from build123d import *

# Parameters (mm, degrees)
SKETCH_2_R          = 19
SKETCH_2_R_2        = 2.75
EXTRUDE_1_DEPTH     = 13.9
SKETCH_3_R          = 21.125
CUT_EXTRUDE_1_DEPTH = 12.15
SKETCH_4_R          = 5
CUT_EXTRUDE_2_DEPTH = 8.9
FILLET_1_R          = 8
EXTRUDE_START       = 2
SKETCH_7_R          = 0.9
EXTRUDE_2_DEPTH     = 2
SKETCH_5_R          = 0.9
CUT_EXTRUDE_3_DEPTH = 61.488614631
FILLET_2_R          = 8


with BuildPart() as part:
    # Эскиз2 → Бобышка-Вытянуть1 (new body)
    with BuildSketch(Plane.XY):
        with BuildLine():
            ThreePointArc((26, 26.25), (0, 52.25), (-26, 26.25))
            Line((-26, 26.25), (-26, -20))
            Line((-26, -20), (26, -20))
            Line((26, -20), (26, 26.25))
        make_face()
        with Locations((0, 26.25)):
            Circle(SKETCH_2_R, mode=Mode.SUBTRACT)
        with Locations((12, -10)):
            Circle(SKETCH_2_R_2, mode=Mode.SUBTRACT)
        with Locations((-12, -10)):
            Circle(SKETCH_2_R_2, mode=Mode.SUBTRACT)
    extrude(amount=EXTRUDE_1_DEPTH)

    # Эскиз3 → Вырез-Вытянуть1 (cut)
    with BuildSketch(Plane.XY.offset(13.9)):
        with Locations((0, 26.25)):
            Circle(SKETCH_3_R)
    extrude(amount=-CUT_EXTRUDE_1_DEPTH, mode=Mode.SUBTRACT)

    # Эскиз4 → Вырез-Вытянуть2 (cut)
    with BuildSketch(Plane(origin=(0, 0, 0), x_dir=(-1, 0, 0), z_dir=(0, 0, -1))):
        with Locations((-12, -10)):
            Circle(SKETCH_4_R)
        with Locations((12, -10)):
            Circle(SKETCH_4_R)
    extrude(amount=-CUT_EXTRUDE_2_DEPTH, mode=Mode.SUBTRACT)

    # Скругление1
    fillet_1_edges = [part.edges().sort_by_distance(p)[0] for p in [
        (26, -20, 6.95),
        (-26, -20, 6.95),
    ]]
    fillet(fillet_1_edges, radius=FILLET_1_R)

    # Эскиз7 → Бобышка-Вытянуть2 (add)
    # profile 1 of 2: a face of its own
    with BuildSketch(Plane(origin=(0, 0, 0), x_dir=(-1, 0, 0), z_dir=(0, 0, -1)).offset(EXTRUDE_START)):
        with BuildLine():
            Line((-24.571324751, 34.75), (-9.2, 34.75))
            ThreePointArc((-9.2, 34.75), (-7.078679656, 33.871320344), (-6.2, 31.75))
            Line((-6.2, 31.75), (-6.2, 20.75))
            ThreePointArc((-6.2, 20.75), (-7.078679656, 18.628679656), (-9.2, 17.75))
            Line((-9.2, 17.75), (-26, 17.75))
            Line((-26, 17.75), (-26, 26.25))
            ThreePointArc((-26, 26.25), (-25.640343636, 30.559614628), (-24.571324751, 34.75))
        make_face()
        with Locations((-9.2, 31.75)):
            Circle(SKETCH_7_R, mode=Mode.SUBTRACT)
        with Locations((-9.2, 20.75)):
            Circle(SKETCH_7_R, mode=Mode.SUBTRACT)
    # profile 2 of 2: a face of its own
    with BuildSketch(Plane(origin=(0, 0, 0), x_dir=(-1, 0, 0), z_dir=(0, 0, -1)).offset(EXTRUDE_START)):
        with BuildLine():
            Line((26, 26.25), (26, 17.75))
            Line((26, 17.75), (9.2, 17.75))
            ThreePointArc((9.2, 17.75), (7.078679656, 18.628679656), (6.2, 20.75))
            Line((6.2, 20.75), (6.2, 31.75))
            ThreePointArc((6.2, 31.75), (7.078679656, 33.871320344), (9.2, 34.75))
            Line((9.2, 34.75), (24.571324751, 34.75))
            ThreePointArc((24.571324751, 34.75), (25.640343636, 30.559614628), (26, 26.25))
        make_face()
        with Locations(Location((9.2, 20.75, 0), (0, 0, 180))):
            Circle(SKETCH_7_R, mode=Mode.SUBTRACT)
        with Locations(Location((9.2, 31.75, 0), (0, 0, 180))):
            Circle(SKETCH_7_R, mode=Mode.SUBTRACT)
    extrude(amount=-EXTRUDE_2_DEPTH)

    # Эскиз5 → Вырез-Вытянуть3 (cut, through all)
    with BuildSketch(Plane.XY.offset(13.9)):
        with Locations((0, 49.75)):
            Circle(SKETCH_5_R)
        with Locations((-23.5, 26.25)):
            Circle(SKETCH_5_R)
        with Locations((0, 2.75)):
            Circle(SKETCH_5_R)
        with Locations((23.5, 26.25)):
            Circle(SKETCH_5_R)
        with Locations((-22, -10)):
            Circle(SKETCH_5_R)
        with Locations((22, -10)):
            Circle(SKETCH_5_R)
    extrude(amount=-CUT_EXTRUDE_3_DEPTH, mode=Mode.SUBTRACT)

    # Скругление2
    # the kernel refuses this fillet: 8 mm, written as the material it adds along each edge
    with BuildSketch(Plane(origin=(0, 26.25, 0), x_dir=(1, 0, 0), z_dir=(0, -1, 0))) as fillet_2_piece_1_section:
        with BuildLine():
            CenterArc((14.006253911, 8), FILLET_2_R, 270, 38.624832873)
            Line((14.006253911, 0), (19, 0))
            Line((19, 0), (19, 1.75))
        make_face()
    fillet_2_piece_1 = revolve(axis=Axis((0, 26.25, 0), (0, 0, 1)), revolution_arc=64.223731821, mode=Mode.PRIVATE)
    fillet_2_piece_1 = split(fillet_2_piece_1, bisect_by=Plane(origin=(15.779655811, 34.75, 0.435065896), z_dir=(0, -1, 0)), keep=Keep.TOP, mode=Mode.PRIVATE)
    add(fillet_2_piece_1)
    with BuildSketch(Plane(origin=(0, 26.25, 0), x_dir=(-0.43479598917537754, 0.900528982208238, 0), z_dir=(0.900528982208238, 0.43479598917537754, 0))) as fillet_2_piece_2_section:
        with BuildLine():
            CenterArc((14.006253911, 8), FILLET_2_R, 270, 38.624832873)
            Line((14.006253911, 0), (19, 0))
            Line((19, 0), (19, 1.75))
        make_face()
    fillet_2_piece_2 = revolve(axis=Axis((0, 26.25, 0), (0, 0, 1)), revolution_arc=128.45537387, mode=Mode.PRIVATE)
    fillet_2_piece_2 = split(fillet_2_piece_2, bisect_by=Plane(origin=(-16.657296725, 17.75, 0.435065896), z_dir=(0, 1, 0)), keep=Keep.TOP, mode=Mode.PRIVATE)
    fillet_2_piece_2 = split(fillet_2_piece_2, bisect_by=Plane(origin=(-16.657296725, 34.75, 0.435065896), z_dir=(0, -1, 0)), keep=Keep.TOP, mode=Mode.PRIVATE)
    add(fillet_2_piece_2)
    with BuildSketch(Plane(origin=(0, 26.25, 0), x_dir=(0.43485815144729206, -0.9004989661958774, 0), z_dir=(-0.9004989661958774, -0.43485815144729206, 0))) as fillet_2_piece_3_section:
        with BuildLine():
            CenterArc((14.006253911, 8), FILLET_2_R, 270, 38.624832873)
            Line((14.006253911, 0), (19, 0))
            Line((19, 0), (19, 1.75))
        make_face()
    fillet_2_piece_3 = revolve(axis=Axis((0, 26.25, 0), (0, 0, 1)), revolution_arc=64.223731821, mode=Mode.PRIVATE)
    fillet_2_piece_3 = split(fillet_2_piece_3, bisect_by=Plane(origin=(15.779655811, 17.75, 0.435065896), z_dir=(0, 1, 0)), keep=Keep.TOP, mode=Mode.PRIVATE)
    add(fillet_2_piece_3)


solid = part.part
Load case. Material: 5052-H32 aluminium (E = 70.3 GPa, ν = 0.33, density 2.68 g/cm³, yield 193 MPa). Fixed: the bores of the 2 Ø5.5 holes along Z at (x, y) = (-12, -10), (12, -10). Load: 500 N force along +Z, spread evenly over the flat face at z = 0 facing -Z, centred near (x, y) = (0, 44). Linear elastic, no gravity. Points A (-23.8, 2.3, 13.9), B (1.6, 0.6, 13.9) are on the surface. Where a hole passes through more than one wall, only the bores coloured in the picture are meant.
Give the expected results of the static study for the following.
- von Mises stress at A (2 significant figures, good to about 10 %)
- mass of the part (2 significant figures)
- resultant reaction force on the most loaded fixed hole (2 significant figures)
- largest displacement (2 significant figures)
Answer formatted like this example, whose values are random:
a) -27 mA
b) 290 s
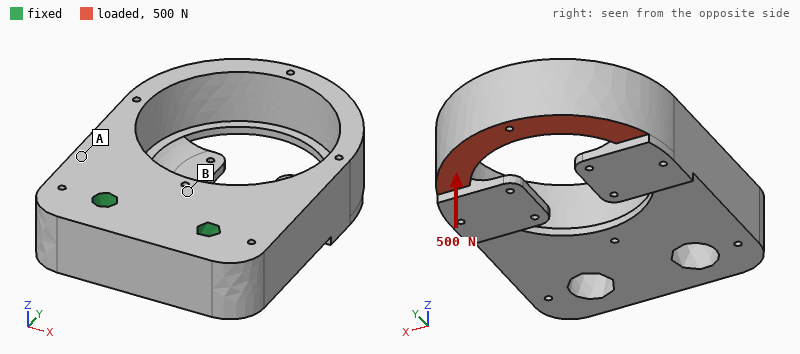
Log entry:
a) 22 MPa
b) 76 g
c) 250 N
d) 0.19 mm
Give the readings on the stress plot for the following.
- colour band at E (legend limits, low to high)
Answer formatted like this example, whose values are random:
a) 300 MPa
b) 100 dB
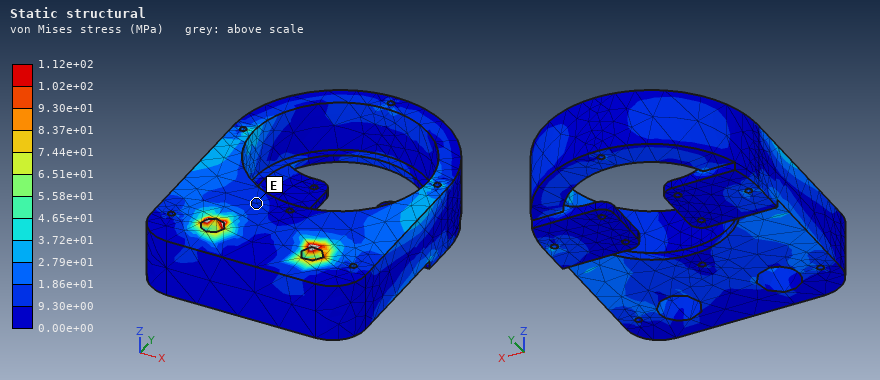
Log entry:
a) 9.30e+00 to 1.86e+01 MPa
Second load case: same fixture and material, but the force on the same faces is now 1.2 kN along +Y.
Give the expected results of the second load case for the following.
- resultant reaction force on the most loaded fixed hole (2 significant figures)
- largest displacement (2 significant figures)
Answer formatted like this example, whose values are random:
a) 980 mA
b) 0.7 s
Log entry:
a) 640 N
b) 0.11 mm
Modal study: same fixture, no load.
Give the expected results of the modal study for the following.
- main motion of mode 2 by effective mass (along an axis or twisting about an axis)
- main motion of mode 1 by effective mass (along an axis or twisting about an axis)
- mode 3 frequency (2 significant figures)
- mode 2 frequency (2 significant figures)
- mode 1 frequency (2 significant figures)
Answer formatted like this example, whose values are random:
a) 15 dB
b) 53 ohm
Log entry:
a) along X
b) along Z
c) 5600 Hz
d) 3900 Hz
e) 2300 Hz
